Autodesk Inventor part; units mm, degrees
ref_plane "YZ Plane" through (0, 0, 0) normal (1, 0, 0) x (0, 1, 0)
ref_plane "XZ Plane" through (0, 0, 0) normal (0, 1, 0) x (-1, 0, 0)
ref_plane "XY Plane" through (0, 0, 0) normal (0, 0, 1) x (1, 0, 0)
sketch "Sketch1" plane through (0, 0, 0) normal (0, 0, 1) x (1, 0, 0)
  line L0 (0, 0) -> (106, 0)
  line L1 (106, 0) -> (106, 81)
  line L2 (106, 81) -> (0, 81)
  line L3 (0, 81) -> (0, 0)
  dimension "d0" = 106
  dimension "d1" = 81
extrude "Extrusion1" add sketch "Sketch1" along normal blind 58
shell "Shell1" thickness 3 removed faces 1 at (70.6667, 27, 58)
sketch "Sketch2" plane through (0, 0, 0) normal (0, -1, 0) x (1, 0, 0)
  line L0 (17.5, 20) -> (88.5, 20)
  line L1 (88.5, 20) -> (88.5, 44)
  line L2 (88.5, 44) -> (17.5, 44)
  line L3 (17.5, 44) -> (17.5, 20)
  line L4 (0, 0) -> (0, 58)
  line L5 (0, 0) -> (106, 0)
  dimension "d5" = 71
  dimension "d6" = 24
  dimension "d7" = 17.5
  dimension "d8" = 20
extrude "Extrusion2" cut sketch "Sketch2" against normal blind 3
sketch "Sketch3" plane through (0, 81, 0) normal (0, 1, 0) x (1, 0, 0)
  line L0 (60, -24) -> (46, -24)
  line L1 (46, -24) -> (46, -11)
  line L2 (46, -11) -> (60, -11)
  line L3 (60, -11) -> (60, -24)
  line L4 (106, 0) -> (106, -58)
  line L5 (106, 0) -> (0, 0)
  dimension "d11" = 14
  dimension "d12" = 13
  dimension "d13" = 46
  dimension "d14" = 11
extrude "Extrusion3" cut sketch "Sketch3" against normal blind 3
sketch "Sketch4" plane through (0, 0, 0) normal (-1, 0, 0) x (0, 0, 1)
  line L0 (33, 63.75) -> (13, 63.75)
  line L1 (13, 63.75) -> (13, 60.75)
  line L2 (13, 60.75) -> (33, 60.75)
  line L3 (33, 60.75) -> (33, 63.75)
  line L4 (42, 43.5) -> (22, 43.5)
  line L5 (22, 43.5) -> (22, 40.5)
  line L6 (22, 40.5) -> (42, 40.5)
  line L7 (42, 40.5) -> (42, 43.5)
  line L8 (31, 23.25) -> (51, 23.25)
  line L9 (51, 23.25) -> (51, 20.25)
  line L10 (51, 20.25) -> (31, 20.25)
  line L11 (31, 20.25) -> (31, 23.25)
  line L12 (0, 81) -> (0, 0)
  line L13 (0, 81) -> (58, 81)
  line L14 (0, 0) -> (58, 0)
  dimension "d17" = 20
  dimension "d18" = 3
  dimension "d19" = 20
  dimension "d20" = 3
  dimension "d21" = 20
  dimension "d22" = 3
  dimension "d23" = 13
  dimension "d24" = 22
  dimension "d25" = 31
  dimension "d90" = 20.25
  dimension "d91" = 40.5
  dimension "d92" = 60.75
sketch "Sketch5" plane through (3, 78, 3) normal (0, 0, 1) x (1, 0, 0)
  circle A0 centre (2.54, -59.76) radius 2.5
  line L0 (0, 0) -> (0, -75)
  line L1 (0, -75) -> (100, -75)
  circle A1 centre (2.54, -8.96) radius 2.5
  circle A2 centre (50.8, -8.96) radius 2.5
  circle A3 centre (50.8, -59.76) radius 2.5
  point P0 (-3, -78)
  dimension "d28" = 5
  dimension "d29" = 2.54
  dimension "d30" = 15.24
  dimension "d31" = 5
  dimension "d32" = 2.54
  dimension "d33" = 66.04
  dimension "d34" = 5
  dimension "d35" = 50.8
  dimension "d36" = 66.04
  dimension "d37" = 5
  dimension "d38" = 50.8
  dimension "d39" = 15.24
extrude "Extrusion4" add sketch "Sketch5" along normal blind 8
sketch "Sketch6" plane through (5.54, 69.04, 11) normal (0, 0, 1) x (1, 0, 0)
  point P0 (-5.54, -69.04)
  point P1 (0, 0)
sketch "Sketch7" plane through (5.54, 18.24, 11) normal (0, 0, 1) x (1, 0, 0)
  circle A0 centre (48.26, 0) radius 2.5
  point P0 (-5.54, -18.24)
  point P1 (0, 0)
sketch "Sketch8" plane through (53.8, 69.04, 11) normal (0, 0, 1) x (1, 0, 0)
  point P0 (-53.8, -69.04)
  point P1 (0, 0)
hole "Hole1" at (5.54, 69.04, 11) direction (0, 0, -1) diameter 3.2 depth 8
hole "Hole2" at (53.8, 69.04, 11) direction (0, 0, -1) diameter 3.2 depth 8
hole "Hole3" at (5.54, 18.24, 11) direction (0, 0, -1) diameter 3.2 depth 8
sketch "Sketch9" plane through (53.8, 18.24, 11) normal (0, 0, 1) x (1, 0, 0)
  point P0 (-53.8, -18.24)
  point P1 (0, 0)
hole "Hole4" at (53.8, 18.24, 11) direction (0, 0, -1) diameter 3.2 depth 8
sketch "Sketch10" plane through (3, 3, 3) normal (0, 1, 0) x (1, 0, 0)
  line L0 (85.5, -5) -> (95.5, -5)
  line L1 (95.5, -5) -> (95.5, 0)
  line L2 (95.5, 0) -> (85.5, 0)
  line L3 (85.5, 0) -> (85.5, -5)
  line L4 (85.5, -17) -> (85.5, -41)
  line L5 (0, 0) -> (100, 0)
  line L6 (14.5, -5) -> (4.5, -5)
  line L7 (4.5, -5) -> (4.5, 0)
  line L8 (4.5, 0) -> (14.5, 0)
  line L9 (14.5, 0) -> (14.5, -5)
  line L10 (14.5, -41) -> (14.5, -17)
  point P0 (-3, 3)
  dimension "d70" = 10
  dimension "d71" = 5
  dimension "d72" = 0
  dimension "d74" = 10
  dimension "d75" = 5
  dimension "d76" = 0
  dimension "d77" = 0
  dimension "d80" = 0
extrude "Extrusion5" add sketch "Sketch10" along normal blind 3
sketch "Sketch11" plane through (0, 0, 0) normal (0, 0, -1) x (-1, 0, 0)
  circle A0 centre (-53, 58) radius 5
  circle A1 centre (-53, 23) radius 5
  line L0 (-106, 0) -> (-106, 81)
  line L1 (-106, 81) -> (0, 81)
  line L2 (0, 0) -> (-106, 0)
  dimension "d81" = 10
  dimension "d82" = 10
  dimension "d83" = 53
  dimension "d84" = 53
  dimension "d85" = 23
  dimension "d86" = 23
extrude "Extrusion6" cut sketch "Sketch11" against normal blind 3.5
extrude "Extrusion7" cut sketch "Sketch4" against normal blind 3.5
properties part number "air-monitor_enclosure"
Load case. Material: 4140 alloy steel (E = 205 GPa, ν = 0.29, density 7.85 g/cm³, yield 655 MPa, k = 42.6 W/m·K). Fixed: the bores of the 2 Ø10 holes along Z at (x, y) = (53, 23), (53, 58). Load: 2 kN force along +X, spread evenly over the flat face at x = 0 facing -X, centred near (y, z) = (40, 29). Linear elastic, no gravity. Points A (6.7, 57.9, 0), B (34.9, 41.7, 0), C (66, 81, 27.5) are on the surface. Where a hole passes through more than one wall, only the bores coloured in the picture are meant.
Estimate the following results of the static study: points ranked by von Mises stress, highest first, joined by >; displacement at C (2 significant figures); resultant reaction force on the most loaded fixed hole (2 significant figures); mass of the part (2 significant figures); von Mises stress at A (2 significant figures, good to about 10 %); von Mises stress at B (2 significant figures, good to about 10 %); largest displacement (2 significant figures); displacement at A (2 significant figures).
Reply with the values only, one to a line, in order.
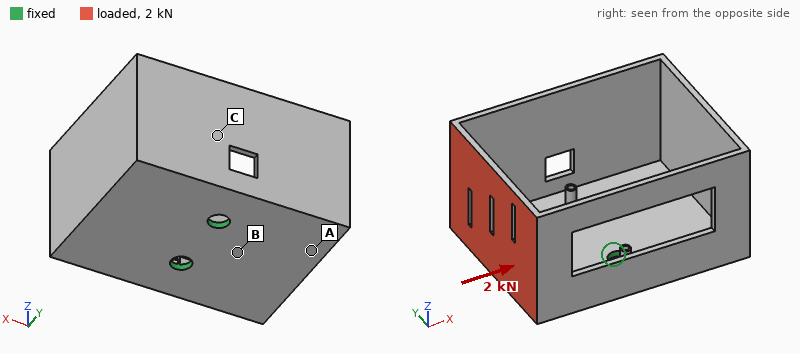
B > A > C
0.20 mm
1.0 kN
620 g
43 MPa
78 MPa
0.67 mm
0.29 mm
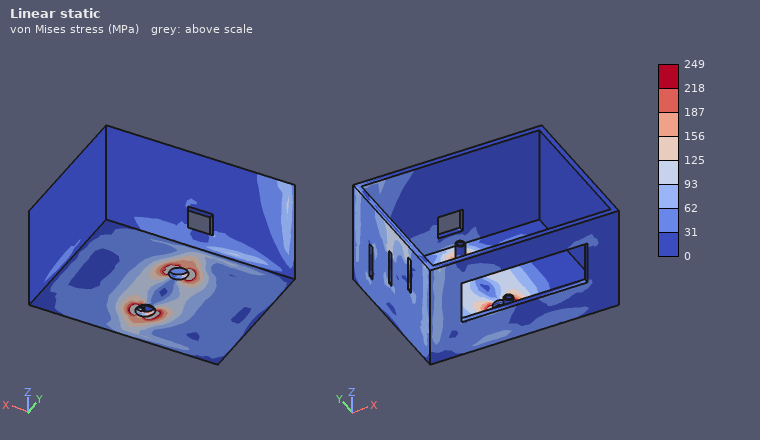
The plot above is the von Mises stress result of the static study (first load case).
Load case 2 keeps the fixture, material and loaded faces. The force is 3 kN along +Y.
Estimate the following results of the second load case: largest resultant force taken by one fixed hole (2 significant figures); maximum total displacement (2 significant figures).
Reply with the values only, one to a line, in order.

4.3 kN
0.62 mm
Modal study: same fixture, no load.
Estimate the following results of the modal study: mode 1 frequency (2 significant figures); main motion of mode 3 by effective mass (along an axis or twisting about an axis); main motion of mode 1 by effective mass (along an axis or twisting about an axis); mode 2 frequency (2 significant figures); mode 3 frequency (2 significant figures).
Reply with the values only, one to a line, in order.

390 Hz
along Y
along X
670 Hz
830 Hz
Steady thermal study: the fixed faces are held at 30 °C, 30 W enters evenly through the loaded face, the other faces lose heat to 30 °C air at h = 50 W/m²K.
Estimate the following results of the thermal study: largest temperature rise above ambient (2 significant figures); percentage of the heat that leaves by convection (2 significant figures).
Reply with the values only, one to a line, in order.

50 K
85 %
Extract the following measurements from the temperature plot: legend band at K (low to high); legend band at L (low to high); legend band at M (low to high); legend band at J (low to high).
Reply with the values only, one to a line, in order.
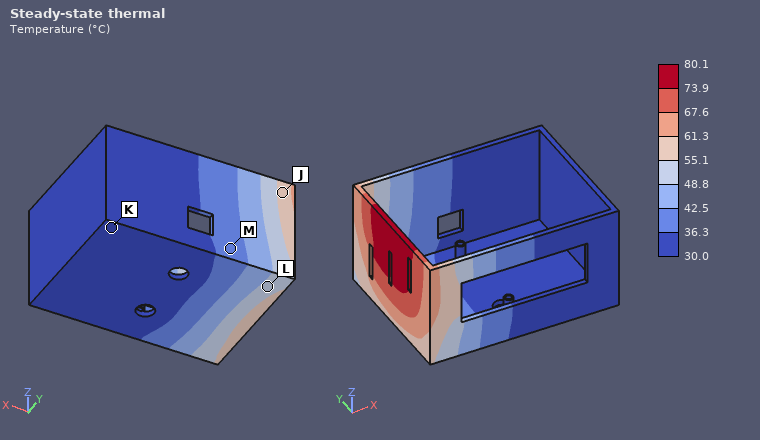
30.0 to 36.3 °C
48.8 to 55.1 °C
36.3 to 42.5 °C
55.1 to 61.3 °C
